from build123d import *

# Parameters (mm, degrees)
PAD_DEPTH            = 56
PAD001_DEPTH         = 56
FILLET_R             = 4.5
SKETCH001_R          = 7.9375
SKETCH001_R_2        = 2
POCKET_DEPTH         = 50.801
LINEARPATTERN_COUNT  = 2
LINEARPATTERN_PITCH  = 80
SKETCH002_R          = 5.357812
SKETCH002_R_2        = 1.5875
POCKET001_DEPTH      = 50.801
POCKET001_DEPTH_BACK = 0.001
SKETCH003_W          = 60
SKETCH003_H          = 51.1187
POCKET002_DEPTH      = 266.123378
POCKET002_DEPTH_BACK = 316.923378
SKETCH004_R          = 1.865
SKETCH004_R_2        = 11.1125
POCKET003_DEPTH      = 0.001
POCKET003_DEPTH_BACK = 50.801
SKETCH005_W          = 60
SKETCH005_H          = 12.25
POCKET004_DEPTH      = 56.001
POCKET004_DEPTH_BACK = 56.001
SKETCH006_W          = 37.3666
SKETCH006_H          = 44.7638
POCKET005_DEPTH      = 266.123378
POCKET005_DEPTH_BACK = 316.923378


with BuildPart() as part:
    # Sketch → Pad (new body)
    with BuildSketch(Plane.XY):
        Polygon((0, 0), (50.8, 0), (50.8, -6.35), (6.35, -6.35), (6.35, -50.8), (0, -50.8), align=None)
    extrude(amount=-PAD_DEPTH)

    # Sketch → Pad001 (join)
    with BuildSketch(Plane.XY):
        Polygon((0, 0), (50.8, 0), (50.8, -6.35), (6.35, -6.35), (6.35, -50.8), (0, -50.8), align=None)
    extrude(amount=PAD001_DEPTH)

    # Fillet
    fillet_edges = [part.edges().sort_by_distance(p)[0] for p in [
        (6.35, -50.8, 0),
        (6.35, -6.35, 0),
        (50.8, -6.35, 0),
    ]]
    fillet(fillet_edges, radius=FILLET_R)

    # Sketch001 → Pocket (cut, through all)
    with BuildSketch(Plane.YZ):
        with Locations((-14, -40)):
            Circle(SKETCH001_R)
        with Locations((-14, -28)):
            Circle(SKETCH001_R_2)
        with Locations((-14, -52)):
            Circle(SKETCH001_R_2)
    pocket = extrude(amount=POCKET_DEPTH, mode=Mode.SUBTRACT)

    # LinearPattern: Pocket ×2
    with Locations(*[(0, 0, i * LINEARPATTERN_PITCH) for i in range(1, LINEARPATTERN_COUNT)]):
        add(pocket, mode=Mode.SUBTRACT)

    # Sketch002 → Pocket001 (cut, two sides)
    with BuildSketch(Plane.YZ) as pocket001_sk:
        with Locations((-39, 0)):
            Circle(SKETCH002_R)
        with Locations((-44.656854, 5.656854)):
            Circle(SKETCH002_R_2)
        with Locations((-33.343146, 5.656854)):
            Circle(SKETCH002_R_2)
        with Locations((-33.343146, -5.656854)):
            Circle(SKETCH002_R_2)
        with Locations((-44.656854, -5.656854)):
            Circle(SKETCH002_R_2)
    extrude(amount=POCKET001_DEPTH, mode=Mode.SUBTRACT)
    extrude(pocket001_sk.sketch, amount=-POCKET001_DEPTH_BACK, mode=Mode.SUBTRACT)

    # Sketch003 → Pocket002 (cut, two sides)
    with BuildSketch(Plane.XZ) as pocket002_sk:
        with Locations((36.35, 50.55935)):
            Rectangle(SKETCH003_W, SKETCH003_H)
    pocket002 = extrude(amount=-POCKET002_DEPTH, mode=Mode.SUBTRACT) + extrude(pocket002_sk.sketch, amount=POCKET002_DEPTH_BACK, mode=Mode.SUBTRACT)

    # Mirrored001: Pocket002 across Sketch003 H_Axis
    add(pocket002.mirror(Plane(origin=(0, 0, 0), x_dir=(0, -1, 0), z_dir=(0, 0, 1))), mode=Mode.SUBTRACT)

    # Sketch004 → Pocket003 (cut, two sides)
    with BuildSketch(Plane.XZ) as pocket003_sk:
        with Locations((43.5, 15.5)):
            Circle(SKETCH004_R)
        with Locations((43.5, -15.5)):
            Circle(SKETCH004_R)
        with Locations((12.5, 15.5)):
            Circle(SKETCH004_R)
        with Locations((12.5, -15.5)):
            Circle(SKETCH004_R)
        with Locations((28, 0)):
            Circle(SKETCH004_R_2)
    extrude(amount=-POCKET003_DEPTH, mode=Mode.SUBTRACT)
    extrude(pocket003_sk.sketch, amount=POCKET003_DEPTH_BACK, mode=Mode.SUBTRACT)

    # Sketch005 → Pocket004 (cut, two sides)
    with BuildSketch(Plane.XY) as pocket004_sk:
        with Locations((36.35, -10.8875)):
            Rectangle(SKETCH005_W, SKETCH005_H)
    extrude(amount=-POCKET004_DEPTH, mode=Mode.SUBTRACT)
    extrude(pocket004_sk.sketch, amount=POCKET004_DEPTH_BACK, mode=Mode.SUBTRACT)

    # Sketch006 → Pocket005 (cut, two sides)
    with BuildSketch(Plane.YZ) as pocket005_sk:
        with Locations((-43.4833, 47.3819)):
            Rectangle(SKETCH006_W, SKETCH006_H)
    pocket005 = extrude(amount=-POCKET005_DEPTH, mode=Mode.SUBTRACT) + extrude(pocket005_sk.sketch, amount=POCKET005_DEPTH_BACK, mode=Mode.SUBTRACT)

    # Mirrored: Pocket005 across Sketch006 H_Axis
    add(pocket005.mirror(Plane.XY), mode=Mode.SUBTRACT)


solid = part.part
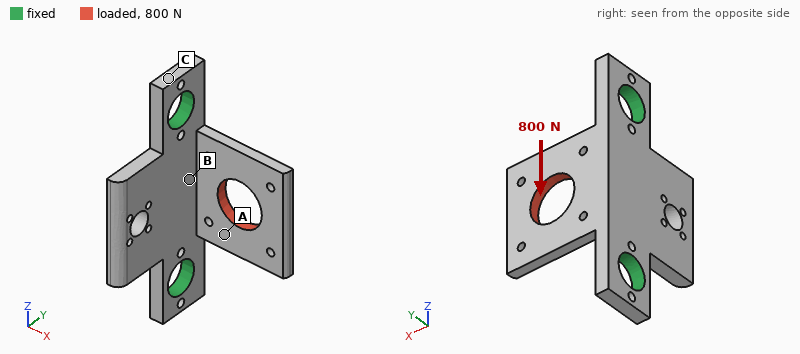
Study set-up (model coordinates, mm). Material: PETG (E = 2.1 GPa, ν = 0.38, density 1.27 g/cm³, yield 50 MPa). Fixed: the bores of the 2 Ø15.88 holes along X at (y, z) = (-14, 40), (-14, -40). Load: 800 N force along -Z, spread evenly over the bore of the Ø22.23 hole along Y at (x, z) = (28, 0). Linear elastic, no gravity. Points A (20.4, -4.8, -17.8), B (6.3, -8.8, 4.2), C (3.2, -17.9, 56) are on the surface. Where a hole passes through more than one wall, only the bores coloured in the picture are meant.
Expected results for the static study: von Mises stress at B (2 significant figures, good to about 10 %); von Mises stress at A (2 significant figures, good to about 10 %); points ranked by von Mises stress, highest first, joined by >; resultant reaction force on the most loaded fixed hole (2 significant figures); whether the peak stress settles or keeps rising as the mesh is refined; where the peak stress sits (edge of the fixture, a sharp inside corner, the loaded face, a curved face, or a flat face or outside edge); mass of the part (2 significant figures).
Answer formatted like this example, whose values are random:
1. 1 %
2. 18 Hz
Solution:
1. 6.3 MPa
2. 9.7 MPa
3. A > B > C
4. 540 N
5. keeps rising
6. a sharp inside corner
7. 39 g
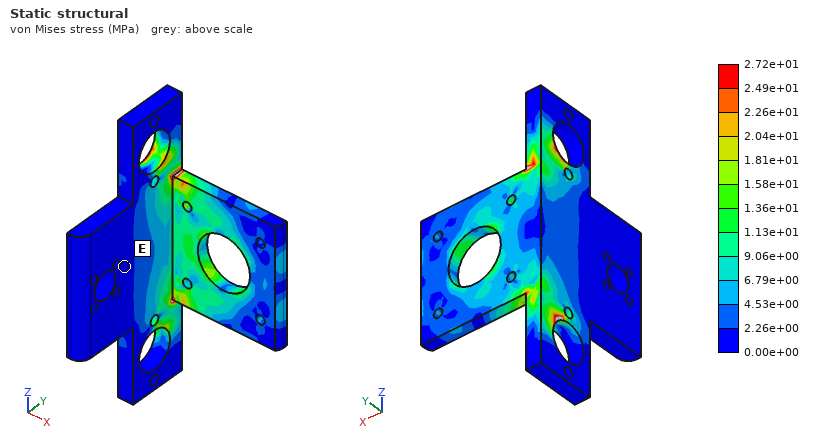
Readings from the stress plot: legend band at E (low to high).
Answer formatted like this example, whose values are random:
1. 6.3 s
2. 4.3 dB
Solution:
1. 0.00e+00 to 2.26e+00 MPa
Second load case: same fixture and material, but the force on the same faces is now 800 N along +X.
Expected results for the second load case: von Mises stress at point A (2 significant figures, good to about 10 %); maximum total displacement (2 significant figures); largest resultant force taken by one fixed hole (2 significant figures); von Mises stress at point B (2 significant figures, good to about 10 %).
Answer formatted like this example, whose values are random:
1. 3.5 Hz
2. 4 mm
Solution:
1. 5.9 MPa
2. 1.4 mm
3. 440 N
4. 2.5 MPa
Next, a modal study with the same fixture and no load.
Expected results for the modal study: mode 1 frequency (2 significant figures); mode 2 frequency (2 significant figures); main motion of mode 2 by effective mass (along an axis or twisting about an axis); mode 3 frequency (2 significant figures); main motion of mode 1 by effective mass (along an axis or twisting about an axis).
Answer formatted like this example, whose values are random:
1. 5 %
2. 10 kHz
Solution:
1. 370 Hz
2. 760 Hz
3. along X
4. 870 Hz
5. along Y
